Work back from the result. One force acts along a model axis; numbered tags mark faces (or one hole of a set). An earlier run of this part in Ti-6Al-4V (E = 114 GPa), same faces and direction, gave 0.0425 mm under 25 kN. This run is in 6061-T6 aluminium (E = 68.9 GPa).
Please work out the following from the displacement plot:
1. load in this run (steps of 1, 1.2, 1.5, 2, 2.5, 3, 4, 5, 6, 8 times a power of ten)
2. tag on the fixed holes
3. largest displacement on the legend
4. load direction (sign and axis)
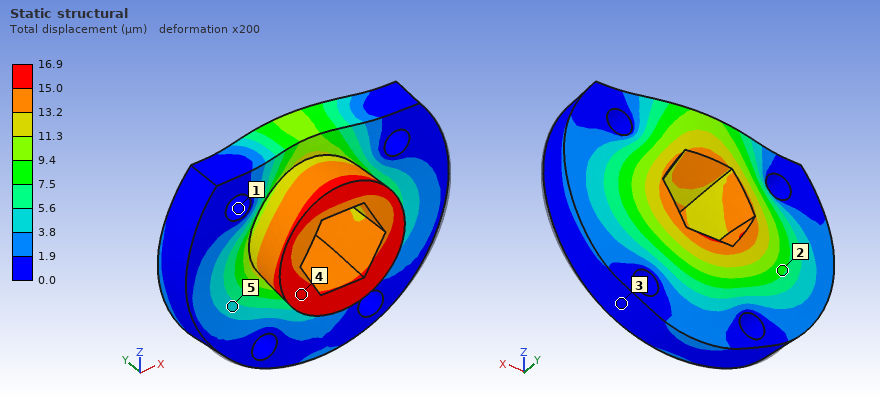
6 kN
1
16.9 µm
+Y
